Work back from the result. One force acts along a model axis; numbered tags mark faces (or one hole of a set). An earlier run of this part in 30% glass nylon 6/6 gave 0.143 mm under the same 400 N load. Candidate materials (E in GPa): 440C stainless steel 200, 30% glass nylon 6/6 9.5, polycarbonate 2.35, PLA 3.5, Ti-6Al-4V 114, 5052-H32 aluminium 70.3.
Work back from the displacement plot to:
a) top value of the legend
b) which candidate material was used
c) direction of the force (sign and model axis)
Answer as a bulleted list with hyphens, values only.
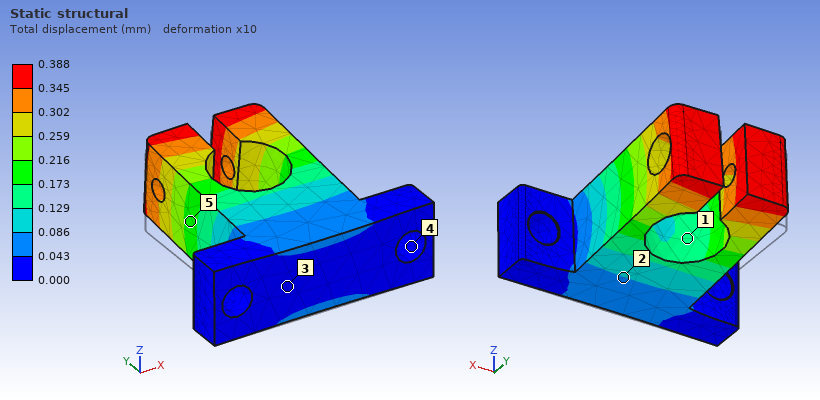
- 0.388 mm
- PLA
- +Z
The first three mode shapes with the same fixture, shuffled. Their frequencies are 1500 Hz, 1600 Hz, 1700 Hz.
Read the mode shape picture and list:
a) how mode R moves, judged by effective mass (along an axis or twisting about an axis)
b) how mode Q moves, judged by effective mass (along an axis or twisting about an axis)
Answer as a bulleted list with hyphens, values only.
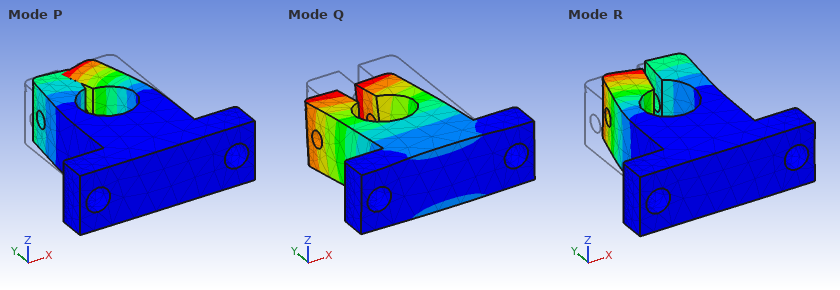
- along X
- along Z
